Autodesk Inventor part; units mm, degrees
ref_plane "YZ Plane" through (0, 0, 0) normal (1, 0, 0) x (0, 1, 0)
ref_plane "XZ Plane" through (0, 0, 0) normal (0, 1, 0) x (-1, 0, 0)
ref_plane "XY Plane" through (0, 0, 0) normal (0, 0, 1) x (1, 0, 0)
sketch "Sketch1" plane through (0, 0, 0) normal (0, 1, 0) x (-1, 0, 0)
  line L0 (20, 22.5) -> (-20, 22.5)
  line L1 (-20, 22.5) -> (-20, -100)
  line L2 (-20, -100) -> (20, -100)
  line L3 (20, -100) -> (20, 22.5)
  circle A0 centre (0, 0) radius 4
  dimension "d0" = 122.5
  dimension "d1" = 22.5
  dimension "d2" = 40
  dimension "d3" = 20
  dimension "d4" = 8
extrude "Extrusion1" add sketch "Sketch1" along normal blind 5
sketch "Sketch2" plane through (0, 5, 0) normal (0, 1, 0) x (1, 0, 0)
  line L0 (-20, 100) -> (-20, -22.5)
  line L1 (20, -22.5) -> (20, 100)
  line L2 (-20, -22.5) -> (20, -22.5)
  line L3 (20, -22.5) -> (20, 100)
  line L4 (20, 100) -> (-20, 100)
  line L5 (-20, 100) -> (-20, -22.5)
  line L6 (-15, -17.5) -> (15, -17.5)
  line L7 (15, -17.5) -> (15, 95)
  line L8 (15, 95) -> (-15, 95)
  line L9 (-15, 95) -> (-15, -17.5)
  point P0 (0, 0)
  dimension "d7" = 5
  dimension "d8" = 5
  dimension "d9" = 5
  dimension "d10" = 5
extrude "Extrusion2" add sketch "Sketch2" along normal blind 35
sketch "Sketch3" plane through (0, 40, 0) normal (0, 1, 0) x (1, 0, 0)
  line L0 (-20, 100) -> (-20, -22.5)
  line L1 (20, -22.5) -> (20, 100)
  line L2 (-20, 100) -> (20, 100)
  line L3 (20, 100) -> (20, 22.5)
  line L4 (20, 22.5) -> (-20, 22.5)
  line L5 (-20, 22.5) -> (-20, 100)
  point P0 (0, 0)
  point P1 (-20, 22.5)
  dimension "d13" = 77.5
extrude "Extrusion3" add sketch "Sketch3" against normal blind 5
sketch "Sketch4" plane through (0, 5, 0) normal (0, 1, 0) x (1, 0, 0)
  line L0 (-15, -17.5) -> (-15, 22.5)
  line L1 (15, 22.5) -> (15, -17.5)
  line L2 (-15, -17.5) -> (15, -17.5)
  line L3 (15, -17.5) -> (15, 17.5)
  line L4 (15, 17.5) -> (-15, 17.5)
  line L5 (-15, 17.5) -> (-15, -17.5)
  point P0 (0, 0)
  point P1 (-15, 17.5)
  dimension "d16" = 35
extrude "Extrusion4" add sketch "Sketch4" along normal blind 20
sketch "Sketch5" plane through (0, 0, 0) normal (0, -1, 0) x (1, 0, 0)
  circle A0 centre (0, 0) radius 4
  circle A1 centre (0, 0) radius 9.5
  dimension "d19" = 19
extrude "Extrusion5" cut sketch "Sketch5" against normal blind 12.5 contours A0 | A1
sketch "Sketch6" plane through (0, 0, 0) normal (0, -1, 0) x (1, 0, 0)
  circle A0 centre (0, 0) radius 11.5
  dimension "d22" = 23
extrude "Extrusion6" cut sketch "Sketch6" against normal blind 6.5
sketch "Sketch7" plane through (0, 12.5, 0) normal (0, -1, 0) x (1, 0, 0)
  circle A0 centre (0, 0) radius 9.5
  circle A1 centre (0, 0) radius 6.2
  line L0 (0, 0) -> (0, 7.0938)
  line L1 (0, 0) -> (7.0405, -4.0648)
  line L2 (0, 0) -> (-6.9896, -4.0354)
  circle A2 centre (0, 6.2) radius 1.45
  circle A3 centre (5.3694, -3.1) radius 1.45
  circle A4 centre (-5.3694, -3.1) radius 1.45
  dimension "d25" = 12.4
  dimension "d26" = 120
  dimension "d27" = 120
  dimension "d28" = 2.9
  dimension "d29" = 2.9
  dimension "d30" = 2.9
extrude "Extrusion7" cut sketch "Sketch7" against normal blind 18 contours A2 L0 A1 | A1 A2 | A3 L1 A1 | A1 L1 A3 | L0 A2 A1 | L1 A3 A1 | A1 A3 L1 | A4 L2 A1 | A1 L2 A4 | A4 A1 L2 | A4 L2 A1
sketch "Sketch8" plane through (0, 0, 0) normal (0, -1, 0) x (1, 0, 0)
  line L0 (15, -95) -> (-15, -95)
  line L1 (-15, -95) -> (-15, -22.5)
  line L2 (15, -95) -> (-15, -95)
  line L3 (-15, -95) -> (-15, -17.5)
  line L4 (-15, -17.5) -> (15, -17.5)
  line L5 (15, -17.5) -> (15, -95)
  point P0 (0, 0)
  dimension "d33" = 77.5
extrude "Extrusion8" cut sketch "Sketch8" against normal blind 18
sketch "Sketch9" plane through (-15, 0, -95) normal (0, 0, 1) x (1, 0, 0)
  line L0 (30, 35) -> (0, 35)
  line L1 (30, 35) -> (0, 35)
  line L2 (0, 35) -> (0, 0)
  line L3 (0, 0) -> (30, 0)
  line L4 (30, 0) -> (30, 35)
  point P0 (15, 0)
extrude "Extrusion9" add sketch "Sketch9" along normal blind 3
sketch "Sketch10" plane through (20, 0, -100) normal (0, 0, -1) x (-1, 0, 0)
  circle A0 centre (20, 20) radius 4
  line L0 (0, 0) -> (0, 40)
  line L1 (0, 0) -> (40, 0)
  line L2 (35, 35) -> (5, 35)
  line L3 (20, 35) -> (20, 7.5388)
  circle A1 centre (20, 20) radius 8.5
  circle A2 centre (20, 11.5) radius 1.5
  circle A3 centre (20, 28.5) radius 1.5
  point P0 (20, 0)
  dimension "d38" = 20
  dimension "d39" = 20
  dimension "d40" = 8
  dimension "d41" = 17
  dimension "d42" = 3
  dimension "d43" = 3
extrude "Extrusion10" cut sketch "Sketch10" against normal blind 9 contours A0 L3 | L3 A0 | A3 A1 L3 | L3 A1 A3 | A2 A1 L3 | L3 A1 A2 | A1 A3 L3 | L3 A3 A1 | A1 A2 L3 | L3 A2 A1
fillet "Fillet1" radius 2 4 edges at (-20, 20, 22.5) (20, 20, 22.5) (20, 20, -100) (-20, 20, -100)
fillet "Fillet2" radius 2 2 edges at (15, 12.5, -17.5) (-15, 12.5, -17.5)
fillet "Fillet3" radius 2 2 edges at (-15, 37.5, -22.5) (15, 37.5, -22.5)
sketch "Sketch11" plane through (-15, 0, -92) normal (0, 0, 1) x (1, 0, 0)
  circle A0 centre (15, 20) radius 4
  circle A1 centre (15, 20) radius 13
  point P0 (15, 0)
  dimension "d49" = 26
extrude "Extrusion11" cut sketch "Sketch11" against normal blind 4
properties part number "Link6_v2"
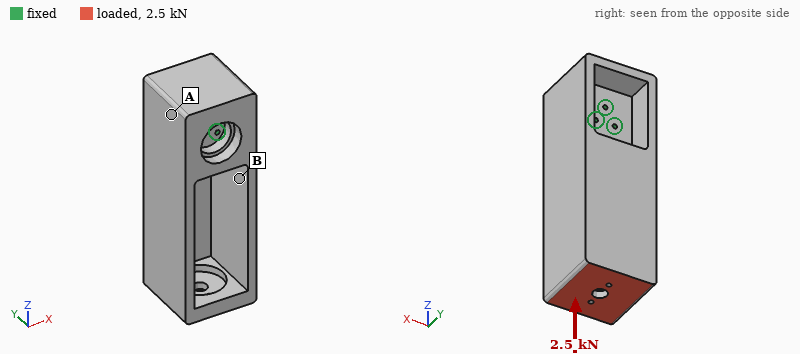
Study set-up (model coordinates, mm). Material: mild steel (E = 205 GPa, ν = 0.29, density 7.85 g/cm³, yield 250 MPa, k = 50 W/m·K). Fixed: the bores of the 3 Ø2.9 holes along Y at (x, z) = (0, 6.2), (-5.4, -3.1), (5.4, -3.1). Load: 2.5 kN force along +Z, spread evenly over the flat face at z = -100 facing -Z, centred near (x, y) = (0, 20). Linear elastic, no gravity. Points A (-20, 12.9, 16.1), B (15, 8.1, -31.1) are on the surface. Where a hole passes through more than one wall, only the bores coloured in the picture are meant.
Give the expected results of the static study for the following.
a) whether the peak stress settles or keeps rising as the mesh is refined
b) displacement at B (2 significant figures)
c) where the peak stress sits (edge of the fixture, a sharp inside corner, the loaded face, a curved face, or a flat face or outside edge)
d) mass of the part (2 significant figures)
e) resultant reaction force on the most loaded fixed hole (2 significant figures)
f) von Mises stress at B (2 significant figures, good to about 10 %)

keeps rising
1.6 µm
a sharp inside corner
740 g
910 N
6.7 MPa
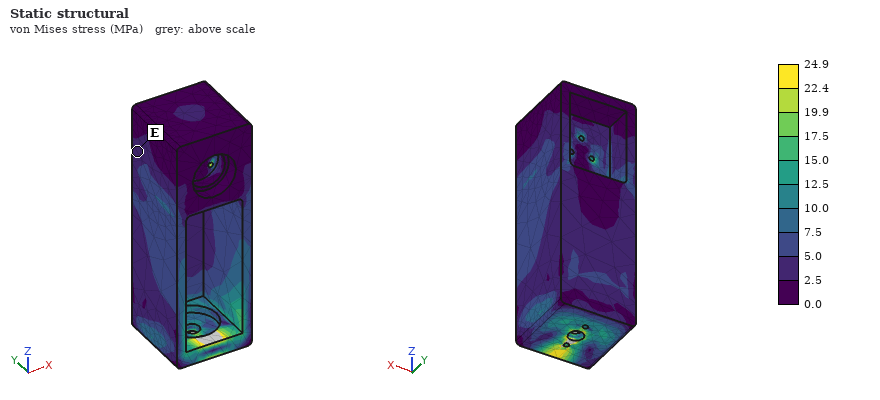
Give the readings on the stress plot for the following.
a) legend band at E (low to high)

2.5 to 5.0 MPa
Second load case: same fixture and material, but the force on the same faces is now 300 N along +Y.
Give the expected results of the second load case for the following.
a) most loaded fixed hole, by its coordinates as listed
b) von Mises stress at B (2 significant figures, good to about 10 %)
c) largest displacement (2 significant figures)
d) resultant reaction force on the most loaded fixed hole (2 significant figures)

(0, 6.2)
5.2 MPa
18 µm
1.0 kN
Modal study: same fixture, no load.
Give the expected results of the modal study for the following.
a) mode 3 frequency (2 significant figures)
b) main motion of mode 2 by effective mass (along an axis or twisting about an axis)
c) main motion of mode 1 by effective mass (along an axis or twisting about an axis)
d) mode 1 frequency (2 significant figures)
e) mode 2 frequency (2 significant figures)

2900 Hz
along Y
along X
1200 Hz
1500 Hz
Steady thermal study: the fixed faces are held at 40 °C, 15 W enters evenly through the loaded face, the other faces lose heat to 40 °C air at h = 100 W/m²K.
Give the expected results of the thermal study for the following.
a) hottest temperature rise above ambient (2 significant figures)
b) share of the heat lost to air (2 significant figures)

19 K
92 %
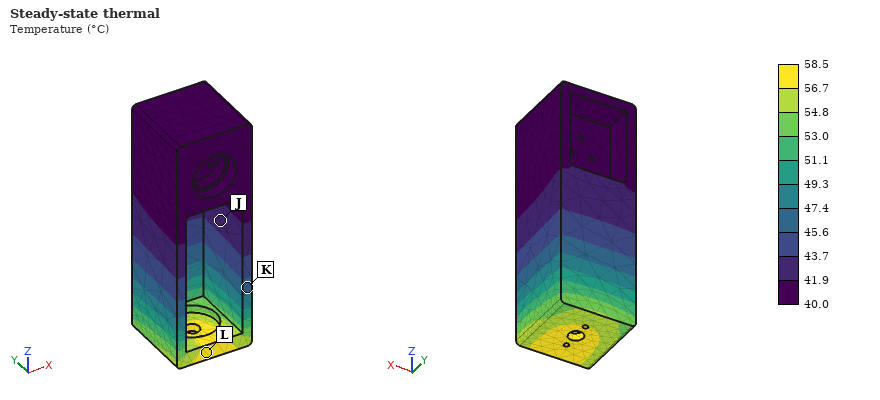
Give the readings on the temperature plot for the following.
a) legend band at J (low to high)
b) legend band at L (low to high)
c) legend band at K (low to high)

41.9 to 43.7 °C
56.7 to 58.5 °C
45.6 to 47.4 °C
